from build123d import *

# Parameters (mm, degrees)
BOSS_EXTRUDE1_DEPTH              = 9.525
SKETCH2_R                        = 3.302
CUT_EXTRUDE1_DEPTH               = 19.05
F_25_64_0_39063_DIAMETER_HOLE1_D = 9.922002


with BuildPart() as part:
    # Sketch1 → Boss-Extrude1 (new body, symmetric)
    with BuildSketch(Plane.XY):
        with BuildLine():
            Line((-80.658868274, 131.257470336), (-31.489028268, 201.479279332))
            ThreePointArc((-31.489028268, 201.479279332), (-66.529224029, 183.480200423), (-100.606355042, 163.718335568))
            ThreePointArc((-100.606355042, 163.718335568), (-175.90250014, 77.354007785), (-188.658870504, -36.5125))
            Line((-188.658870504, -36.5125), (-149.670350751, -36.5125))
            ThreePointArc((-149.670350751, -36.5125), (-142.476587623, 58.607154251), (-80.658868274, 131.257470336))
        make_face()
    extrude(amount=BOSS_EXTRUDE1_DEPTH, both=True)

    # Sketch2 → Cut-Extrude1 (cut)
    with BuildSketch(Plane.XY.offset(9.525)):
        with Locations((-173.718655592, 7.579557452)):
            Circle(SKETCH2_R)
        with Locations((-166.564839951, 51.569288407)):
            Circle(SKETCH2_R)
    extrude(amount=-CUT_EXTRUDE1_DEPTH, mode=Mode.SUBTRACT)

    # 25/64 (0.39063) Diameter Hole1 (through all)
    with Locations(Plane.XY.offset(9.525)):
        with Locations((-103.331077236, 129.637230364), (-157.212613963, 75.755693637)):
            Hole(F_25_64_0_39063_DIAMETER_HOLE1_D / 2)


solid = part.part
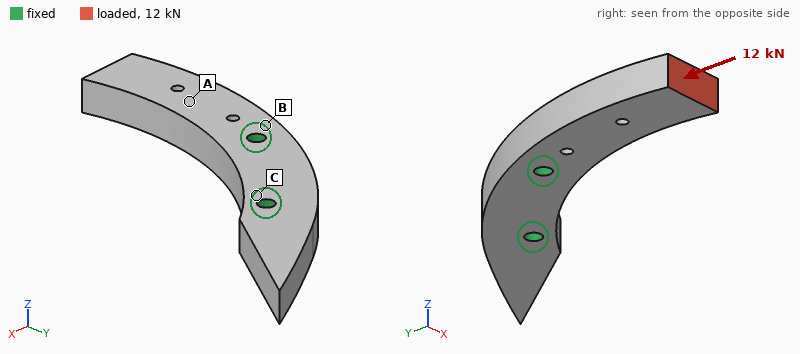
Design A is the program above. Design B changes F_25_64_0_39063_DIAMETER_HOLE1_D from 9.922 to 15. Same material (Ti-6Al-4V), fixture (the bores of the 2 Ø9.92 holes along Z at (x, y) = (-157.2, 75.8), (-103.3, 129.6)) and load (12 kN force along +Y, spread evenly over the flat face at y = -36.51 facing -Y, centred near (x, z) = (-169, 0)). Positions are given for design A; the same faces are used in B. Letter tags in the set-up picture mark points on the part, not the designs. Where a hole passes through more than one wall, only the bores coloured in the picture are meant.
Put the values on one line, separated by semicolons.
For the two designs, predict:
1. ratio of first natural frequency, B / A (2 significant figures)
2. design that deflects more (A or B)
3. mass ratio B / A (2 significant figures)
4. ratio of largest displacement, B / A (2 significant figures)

1.1; A; 0.98; 0.77
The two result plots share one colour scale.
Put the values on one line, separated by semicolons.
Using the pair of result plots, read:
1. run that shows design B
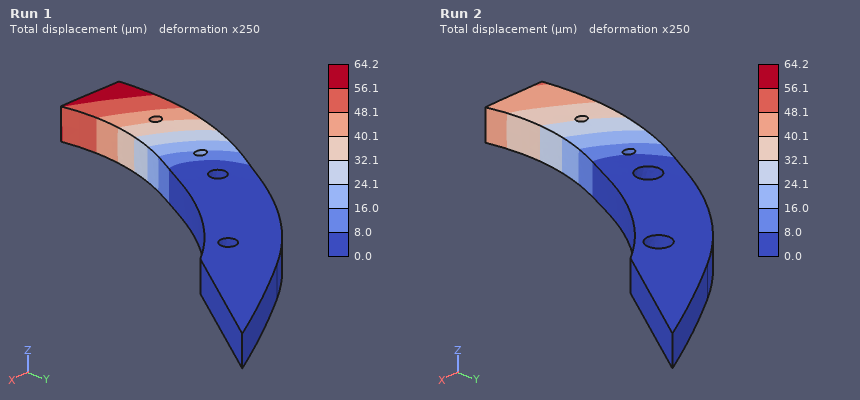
Run 2
